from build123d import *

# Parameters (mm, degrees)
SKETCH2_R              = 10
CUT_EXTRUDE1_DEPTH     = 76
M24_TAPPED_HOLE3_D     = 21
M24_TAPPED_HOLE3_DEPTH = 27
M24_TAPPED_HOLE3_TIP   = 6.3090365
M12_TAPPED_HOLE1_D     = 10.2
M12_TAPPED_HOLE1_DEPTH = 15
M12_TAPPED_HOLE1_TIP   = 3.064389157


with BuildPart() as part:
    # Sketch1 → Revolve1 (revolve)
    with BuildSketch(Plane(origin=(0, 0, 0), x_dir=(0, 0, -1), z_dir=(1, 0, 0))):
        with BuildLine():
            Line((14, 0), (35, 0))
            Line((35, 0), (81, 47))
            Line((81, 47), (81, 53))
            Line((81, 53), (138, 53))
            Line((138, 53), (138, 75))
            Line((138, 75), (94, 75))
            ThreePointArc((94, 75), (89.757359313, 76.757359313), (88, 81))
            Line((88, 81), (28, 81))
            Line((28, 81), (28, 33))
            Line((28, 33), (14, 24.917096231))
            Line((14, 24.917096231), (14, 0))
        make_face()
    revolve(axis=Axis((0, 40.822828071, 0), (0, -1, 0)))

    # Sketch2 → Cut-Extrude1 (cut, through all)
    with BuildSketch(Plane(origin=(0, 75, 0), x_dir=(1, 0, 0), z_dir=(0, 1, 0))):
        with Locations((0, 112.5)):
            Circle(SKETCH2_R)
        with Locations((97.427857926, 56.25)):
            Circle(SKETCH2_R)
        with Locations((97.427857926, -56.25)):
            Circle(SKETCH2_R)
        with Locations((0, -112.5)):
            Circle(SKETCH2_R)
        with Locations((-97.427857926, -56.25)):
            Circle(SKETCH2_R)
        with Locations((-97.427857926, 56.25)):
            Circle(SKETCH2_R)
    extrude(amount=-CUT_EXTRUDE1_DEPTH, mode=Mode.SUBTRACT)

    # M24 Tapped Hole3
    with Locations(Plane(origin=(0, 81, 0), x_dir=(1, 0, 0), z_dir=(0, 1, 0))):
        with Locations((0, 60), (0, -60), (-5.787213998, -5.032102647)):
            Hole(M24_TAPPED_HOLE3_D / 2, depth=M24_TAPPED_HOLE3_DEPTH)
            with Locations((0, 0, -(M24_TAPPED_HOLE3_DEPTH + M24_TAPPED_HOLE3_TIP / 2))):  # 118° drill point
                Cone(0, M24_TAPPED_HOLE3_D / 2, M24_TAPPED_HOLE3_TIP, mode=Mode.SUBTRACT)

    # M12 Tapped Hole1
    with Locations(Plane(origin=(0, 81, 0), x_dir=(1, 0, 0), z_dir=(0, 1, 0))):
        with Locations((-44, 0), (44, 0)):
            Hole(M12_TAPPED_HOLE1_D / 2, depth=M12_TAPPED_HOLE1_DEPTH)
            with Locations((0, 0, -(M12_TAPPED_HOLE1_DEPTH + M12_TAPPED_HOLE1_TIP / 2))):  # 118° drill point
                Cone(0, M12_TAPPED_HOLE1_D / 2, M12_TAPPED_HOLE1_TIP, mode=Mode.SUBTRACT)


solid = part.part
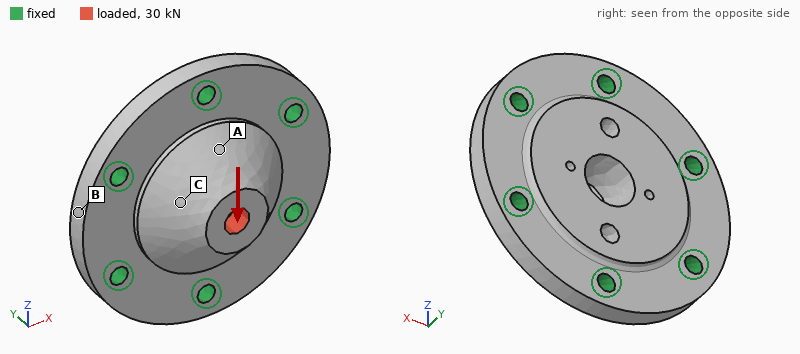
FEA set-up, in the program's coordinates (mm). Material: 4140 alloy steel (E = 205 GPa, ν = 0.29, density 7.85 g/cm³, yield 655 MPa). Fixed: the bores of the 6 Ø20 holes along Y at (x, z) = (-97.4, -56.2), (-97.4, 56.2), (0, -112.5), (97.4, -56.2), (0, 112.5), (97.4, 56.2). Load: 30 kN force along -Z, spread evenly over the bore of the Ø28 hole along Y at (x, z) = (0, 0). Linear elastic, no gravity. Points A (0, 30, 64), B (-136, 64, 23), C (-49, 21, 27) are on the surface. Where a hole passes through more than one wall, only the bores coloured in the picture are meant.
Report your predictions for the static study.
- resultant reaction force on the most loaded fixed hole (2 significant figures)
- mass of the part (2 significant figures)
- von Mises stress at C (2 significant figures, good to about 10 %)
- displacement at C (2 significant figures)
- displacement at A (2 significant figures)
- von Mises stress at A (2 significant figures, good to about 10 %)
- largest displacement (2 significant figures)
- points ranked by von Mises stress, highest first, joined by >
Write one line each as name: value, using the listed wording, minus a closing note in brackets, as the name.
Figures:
resultant reaction force on the most loaded fixed hole: 8.8 kN
mass of the part: 15 kg
von Mises stress at C: 4.4 MPa
displacement at C: 3.4 µm
displacement at A: 3.9 µm
von Mises stress at A: 8.1 MPa
largest displacement: 7.5 µm
points ranked by von Mises stress, highest first, joined by >: A > C > B
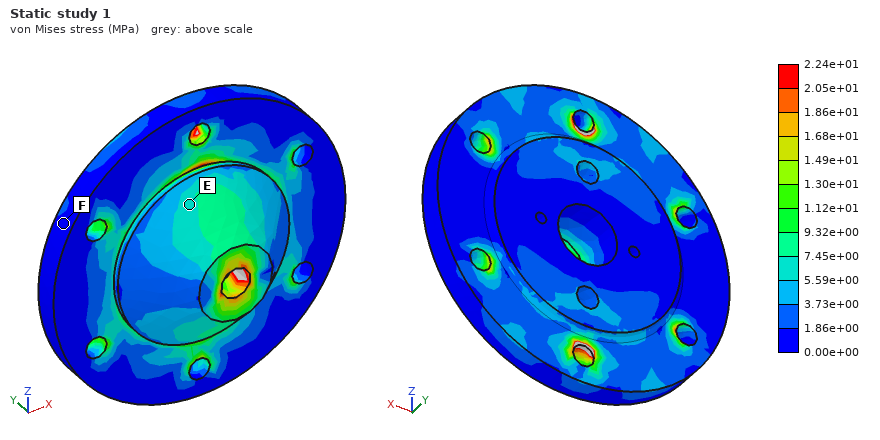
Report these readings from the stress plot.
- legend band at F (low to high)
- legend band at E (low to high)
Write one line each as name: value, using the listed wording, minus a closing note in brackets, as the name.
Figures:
legend band at F: 0.00e+00 to 1.86e+00 MPa
legend band at E: 5.59e+00 to 7.45e+00 MPa
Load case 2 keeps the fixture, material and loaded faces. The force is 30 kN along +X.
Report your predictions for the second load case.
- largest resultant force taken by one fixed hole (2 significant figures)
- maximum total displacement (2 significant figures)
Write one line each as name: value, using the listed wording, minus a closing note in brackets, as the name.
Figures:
largest resultant force taken by one fixed hole: 7.8 kN
maximum total displacement: 7.3 µm
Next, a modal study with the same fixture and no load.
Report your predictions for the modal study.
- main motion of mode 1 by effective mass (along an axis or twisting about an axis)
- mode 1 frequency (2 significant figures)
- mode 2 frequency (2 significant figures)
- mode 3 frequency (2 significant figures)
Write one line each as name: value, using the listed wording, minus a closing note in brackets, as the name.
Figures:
main motion of mode 1 by effective mass: along Y
mode 1 frequency: 4400 Hz
mode 2 frequency: 6200 Hz
mode 3 frequency: 6200 Hz
